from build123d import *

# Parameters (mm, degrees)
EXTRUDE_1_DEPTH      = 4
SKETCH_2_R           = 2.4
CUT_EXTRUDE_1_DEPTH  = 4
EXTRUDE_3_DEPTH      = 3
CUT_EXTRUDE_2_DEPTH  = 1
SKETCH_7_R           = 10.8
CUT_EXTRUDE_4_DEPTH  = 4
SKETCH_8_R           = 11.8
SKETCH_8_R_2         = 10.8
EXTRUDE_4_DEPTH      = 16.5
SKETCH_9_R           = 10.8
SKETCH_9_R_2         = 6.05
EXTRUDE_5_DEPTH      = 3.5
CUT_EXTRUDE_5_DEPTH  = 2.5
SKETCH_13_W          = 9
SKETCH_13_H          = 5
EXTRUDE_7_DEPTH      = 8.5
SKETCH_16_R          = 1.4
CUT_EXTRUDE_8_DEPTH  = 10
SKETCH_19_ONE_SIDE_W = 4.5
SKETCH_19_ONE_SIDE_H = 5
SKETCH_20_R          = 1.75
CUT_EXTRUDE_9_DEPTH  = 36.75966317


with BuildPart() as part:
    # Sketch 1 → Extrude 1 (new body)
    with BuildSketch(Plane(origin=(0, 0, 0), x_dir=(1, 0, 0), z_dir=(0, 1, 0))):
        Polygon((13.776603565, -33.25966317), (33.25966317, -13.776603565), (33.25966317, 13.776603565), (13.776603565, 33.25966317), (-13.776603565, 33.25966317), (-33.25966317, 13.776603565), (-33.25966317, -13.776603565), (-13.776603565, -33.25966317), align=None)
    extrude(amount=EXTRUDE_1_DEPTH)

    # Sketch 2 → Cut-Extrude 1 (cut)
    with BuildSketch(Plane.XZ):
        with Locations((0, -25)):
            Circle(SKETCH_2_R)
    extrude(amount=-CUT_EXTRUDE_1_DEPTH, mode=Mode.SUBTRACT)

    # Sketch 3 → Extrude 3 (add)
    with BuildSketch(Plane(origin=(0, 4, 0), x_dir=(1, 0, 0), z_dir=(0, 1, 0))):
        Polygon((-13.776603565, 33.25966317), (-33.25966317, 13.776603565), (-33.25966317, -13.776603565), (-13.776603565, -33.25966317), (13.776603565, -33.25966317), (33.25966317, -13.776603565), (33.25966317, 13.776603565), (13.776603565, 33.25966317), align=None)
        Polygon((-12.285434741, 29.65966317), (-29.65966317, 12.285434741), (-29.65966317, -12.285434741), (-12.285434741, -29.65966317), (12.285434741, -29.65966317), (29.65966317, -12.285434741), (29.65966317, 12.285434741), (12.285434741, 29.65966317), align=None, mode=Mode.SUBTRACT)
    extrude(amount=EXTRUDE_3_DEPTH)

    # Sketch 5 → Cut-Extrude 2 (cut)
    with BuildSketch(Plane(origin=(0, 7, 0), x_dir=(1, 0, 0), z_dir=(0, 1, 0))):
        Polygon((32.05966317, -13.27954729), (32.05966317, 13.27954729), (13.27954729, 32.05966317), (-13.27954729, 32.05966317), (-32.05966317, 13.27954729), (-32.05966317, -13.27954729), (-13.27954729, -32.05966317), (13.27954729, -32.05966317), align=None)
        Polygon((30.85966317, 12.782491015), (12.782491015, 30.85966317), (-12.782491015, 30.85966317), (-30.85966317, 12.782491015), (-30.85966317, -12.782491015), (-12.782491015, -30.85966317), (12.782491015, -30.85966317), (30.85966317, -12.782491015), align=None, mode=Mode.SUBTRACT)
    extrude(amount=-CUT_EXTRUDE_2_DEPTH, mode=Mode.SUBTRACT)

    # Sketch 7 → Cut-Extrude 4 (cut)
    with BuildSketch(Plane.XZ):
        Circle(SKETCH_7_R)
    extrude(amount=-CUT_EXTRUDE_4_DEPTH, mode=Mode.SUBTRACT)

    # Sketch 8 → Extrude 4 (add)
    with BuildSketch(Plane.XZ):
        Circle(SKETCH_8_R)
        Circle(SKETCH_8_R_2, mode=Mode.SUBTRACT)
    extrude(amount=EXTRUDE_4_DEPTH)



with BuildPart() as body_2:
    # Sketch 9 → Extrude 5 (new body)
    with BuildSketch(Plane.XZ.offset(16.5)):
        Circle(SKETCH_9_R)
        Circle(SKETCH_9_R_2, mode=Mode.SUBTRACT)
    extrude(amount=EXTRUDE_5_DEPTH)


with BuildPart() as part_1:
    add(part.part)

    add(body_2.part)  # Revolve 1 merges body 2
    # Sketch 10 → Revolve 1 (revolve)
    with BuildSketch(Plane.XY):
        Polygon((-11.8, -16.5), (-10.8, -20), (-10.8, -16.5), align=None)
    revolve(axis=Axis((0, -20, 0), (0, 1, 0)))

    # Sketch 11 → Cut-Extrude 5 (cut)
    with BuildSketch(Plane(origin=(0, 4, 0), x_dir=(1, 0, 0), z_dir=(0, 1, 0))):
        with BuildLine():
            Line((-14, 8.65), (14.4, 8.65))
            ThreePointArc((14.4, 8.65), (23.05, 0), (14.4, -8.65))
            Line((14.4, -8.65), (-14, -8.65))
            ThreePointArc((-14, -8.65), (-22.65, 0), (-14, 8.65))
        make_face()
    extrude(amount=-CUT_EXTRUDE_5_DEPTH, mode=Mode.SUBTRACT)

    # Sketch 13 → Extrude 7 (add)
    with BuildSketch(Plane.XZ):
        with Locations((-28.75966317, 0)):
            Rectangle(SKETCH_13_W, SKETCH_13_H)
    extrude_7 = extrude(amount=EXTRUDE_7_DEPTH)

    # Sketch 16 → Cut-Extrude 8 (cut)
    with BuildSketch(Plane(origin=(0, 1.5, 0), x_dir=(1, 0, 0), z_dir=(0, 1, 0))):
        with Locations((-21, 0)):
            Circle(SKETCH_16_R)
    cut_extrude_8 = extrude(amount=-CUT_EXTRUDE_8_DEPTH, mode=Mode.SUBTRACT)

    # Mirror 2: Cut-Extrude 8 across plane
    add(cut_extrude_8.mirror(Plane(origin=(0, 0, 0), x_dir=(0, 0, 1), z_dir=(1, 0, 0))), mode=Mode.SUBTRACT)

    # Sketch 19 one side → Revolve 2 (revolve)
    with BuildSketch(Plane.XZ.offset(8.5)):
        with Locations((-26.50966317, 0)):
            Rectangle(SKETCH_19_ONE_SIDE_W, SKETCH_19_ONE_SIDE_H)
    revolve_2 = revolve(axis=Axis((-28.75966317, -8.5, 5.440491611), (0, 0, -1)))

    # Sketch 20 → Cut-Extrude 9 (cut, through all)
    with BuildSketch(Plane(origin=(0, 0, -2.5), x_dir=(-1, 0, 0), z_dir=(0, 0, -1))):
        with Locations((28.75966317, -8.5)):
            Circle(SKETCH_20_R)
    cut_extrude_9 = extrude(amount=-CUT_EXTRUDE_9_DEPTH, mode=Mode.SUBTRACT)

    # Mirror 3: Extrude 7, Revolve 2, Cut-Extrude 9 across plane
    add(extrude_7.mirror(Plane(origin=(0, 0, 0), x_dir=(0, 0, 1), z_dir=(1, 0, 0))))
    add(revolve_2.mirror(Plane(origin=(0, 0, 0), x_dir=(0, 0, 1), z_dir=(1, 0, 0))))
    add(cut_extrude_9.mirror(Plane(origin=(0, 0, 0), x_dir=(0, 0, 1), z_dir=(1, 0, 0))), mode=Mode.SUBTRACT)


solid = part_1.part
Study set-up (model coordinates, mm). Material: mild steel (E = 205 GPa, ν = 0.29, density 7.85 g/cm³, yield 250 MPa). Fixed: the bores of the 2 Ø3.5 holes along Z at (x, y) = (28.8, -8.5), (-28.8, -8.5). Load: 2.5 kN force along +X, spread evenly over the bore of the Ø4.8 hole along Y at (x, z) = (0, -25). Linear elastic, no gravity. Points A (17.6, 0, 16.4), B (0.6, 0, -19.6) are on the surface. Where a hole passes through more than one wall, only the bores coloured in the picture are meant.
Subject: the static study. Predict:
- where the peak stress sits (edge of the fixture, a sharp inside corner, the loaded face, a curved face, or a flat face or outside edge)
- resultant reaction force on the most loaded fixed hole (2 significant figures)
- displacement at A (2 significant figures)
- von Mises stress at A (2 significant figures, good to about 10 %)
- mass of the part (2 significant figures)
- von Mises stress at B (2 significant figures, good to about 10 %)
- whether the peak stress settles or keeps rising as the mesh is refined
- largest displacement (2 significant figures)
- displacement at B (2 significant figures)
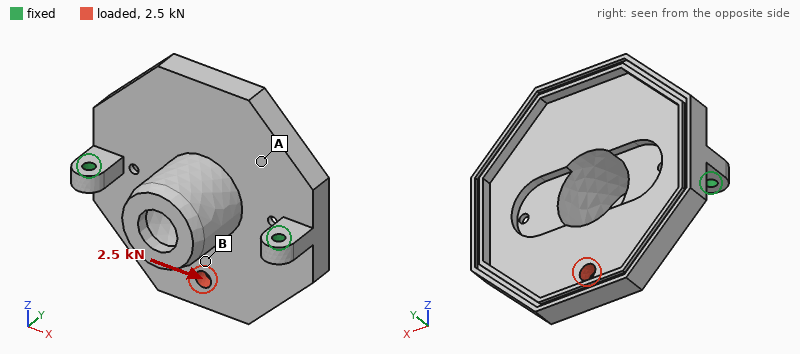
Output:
edge of the fixture
1.6 kN
9.3 µm
18 MPa
140 g
54 MPa
keeps rising
35 µm
26 µm
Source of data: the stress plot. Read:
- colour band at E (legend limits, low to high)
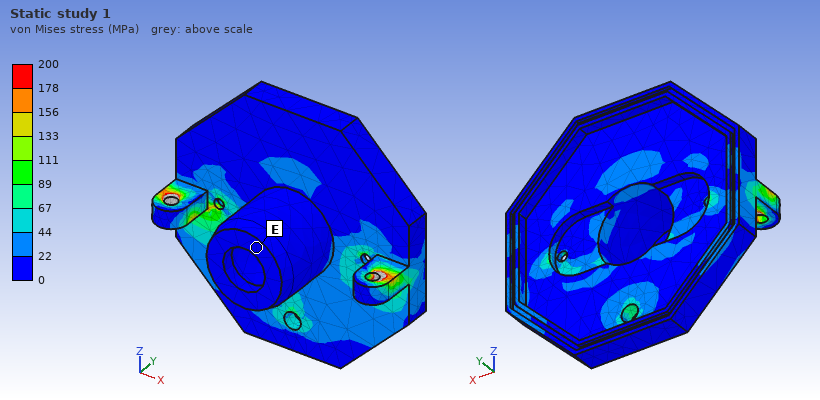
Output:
0 to 22 MPa
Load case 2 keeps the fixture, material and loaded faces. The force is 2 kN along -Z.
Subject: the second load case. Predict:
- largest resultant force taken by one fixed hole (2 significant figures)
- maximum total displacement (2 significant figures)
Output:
1.0 kN
0.10 mm
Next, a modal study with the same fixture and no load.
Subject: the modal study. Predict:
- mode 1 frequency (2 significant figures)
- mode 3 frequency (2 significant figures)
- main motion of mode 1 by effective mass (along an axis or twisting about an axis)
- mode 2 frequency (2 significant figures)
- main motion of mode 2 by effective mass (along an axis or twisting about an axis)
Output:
1300 Hz
4700 Hz
twisting about X
2800 Hz
along Y
